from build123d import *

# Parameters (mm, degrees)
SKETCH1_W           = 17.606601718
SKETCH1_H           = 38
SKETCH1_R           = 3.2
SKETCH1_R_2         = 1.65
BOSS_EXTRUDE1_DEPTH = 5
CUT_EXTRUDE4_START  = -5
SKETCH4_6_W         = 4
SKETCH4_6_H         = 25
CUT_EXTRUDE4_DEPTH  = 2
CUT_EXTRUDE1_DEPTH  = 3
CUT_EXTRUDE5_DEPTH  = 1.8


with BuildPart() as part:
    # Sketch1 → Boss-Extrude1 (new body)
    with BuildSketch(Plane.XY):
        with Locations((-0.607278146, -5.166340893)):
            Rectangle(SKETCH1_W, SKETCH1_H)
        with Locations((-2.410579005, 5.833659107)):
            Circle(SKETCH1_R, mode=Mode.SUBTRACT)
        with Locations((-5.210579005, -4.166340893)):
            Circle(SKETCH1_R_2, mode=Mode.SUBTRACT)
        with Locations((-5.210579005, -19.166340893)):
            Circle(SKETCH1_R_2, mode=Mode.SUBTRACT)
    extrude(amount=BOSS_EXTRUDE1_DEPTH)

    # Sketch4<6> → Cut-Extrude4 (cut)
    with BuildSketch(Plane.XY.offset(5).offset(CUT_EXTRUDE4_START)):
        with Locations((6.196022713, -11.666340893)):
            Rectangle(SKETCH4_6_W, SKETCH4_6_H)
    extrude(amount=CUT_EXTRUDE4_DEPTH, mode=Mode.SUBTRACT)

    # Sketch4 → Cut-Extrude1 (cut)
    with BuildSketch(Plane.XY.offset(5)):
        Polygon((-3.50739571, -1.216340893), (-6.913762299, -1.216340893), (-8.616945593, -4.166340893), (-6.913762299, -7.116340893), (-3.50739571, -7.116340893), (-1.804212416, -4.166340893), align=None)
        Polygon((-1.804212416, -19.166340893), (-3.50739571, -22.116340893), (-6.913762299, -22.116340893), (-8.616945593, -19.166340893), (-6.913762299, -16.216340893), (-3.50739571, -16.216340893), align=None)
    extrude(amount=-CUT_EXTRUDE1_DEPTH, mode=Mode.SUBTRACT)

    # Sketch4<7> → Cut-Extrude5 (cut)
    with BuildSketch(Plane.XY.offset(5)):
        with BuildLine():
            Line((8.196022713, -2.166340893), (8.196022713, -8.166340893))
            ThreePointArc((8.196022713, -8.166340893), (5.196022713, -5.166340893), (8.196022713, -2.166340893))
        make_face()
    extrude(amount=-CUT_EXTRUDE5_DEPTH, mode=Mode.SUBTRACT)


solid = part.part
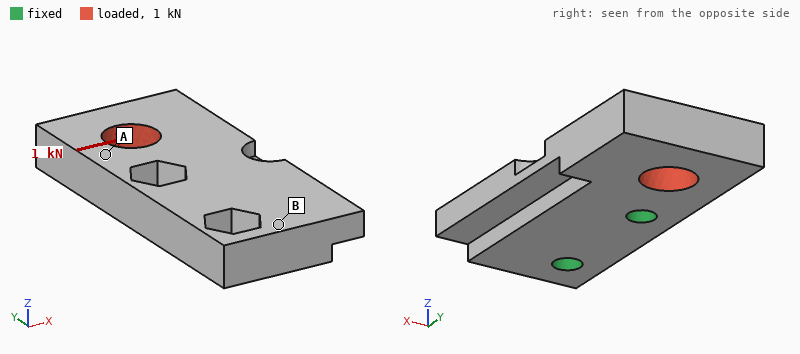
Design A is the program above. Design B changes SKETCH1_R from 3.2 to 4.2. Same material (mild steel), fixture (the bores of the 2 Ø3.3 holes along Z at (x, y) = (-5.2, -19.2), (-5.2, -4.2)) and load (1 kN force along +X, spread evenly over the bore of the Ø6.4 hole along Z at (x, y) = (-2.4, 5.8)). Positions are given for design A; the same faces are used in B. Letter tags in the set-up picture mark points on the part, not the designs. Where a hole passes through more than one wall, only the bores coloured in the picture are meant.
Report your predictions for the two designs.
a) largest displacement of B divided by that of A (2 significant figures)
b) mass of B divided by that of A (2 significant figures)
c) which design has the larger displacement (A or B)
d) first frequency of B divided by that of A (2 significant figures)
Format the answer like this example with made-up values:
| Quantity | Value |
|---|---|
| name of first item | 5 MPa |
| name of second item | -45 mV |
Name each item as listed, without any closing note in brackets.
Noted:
| Quantity | Value |
|---|---|
| largest displacement of B divided by that of A | 1.1 |
| mass of B divided by that of A | 0.96 |
| which design has the larger displacement | B |
| first frequency of B divided by that of A | 1.00 |
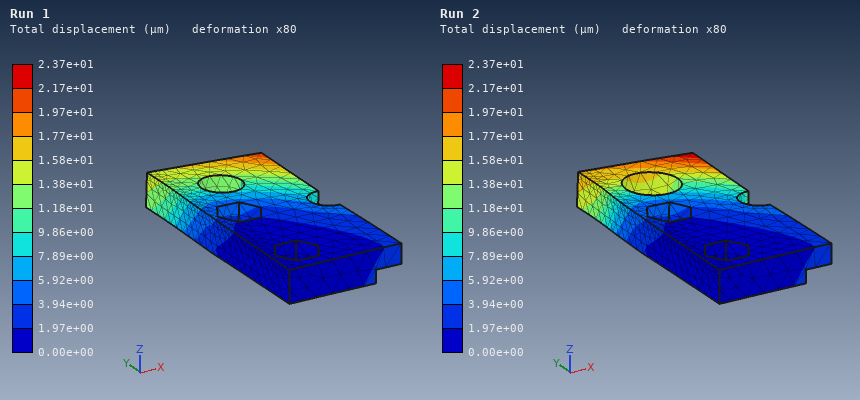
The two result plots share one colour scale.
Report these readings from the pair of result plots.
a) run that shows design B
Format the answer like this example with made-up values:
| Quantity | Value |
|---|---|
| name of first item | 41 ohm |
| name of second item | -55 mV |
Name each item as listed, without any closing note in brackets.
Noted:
| Quantity | Value |
|---|---|
| run that shows design B | Run 2 |
